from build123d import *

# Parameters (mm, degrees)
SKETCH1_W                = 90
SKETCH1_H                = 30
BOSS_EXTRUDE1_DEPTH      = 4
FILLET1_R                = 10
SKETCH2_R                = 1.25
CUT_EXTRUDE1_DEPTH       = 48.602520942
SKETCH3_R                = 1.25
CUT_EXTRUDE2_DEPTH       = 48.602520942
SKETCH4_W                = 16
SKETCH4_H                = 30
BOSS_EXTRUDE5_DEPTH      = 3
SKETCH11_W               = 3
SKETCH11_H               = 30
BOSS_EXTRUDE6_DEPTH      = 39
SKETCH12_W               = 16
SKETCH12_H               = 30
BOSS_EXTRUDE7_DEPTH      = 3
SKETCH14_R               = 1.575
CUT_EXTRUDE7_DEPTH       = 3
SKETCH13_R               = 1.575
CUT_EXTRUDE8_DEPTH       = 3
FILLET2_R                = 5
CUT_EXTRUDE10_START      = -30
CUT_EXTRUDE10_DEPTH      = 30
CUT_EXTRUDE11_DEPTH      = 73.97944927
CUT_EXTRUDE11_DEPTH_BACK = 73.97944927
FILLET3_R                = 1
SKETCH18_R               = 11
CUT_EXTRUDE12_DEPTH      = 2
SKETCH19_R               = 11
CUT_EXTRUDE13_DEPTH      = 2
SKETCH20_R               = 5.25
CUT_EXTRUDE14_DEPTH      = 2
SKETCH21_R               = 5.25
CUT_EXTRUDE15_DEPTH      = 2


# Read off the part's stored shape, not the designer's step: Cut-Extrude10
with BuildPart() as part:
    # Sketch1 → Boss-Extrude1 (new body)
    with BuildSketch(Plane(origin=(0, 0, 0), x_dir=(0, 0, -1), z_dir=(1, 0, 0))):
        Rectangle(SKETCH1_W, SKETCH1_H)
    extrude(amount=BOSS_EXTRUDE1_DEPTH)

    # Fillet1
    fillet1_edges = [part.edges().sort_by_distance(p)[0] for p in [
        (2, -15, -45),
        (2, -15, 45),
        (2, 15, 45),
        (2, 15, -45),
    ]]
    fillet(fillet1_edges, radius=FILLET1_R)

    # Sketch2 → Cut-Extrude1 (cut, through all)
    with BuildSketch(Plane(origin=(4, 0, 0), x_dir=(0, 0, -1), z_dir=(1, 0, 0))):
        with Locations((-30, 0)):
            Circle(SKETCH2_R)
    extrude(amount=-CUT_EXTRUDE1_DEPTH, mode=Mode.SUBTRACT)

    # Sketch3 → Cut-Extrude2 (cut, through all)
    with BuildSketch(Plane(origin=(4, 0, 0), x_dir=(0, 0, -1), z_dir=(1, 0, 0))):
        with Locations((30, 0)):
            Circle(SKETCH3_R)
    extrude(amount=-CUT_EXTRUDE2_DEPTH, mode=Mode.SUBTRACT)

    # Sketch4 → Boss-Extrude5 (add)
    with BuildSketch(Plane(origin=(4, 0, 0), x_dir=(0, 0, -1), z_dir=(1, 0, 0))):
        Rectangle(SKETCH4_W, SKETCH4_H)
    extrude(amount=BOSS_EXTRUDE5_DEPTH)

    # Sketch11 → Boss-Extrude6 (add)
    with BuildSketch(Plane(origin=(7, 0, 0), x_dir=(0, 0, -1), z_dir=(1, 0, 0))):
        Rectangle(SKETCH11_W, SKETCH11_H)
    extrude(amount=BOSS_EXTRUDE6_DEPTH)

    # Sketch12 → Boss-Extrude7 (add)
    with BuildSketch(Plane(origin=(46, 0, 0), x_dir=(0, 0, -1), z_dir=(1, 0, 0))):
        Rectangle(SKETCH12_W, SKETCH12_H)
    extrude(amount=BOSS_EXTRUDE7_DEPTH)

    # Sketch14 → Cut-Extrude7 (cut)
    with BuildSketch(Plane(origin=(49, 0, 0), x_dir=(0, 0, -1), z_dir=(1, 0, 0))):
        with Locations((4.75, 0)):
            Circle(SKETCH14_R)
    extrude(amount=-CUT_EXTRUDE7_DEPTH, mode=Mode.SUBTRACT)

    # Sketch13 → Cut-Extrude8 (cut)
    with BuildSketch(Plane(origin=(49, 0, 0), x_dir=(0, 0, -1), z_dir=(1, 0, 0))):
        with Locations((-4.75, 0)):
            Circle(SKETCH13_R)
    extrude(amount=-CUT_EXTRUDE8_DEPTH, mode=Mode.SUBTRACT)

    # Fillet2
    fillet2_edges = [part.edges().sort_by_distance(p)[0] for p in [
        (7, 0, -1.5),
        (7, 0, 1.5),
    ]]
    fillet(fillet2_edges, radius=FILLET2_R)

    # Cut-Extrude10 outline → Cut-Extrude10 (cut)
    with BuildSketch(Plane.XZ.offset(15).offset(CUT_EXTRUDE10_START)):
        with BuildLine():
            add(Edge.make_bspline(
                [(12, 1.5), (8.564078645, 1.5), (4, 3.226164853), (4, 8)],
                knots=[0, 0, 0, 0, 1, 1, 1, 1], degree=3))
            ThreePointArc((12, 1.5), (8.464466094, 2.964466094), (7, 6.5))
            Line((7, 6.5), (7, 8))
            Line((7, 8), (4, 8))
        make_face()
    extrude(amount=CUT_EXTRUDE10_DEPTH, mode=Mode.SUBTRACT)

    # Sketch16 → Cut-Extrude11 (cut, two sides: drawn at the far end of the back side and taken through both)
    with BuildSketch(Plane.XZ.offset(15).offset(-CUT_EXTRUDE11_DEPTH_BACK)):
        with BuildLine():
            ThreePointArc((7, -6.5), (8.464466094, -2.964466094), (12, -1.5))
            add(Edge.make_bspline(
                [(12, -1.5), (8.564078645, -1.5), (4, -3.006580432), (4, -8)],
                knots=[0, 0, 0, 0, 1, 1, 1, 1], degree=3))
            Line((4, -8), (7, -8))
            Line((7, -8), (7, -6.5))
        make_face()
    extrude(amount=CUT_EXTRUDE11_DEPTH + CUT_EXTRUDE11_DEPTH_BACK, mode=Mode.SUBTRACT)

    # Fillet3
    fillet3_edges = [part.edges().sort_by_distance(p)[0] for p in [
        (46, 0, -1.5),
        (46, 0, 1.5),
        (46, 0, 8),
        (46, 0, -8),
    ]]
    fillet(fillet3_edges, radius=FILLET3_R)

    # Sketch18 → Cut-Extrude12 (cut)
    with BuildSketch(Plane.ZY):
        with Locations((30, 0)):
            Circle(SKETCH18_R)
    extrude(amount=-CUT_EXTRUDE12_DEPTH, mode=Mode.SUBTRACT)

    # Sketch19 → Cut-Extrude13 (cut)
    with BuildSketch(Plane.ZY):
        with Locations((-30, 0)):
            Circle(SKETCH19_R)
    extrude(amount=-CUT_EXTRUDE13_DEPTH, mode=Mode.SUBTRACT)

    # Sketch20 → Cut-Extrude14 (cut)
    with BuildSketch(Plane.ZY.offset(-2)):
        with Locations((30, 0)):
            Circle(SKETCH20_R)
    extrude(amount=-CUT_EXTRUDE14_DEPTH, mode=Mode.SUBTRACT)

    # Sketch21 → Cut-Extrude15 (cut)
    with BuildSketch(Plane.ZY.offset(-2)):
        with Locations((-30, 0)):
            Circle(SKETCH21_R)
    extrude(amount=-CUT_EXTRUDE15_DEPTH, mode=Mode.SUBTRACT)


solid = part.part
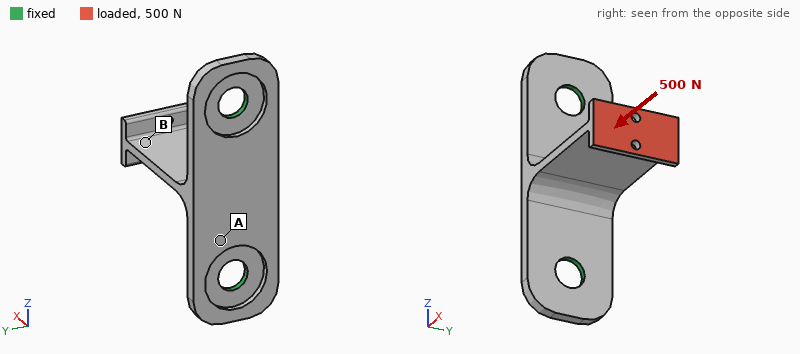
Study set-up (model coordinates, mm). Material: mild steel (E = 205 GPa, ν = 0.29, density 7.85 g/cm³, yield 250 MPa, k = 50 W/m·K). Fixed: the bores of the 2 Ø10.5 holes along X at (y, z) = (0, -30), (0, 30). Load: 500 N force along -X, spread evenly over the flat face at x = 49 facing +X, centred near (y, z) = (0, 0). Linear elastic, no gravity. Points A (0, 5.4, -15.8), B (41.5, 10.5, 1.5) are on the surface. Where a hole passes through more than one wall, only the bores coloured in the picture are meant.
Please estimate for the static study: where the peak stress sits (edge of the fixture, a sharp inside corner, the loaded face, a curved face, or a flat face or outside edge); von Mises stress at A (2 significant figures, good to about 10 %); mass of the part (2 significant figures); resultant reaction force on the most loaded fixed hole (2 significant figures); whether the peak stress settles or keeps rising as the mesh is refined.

edge of the fixture
16 MPa
110 g
440 N
keeps rising
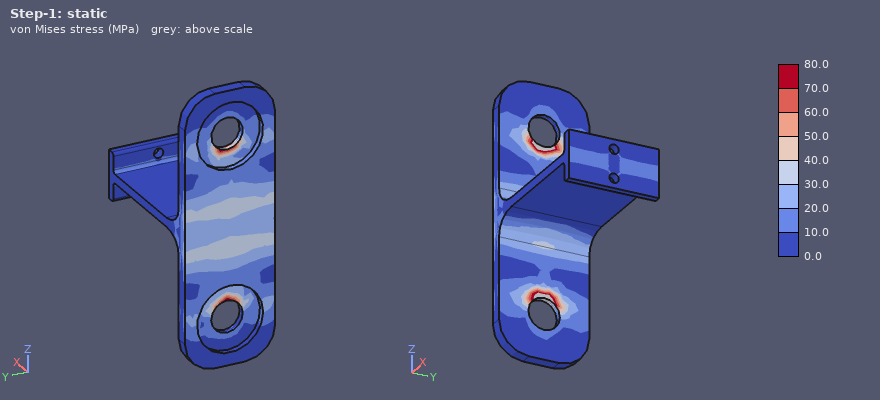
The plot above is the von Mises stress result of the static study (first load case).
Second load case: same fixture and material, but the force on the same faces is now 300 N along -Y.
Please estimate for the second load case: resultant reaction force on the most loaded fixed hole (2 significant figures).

150 N
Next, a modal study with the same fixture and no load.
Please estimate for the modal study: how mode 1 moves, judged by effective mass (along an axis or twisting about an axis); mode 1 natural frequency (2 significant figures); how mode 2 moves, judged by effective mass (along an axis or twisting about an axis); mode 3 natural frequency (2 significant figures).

along Z
980 Hz
along Y
3200 Hz
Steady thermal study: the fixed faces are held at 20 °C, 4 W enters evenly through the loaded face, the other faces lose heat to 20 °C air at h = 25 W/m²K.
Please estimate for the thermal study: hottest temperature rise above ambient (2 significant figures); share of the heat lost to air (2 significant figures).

32 K
50 %
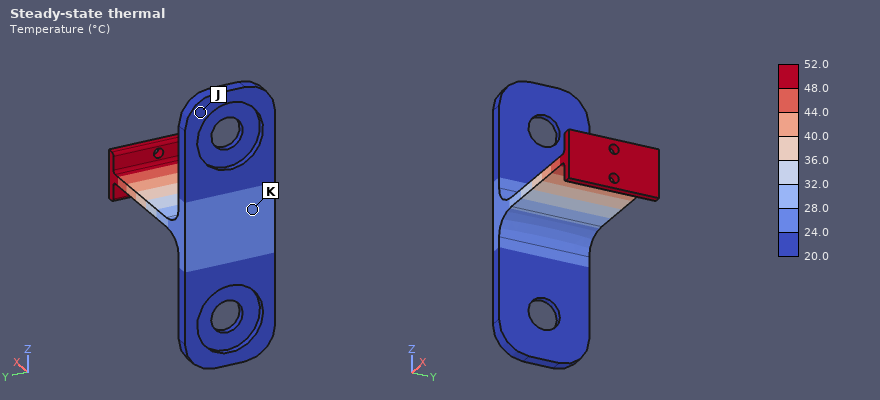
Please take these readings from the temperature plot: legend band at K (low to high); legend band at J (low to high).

24.0 to 28.0 °C
20.0 to 24.0 °C
